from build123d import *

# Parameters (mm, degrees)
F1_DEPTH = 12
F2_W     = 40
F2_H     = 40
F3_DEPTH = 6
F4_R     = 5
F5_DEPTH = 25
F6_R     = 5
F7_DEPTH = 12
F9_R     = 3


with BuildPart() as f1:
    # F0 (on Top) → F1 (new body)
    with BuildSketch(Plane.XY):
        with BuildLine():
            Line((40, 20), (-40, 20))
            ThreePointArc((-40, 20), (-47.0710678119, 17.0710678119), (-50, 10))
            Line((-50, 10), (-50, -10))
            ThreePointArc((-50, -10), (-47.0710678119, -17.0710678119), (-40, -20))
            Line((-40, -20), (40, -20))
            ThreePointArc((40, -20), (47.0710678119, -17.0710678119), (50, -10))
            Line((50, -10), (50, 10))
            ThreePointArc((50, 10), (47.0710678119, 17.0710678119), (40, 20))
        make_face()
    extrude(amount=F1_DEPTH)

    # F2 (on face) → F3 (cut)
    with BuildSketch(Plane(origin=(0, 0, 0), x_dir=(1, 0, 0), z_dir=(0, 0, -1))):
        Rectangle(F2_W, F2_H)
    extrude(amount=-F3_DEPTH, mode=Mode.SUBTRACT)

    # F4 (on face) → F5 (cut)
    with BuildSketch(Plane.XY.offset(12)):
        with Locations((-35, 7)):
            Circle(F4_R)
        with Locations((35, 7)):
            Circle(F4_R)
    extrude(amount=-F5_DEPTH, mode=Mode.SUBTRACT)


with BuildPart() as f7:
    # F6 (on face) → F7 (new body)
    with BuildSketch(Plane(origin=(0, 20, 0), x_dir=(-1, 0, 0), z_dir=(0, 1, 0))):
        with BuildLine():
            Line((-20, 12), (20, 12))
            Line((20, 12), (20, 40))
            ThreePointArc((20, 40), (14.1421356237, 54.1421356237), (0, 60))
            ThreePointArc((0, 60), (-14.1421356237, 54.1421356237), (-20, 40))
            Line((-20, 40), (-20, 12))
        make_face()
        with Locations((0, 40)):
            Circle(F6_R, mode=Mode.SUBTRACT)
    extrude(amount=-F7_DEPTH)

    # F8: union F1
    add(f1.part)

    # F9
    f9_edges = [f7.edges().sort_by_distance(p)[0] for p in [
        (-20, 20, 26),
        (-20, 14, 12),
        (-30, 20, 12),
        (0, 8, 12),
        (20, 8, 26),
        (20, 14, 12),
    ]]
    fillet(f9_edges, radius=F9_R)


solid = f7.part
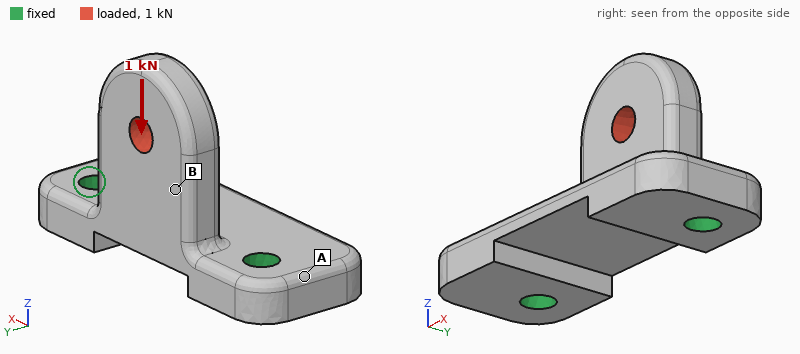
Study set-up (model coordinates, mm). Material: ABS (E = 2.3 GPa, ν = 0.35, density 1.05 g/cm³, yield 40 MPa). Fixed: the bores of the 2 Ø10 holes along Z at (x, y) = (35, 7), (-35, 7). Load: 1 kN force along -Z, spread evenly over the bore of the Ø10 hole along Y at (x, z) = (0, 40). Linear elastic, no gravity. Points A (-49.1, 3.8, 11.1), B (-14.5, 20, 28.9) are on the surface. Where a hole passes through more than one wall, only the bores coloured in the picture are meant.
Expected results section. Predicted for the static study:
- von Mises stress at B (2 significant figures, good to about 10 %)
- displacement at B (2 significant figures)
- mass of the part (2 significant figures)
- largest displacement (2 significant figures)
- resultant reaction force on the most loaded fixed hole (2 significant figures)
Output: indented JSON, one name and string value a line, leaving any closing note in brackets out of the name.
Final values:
{
  "von Mises stress at B": "2.6 MPa",
  "displacement at B": "0.23 mm",
  "mass of the part": "58 g",
  "largest displacement": "0.40 mm",
  "resultant reaction force on the most loaded fixed hole": "620 N"
}
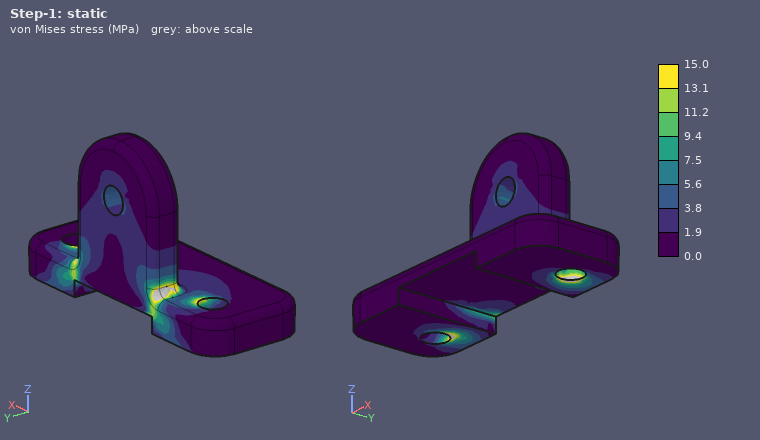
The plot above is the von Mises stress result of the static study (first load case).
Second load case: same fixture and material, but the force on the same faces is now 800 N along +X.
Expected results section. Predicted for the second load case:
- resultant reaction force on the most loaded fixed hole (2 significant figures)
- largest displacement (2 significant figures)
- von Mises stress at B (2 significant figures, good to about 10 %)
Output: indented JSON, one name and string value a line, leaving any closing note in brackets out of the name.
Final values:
{
  "resultant reaction force on the most loaded fixed hole": "690 N",
  "largest displacement": "0.42 mm",
  "von Mises stress at B": "2.5 MPa"
}
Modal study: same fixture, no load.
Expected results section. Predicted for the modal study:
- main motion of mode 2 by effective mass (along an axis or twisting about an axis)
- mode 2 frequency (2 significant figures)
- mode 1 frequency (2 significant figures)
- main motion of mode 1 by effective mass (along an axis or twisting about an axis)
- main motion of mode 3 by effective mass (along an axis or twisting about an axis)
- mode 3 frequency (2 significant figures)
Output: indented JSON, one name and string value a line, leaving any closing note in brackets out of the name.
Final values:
{
  "main motion of mode 2 by effective mass": "along X",
  "mode 2 frequency": "2000 Hz",
  "mode 1 frequency": "760 Hz",
  "main motion of mode 1 by effective mass": "along Y",
  "main motion of mode 3 by effective mass": "along Z",
  "mode 3 frequency": "2700 Hz"
}
